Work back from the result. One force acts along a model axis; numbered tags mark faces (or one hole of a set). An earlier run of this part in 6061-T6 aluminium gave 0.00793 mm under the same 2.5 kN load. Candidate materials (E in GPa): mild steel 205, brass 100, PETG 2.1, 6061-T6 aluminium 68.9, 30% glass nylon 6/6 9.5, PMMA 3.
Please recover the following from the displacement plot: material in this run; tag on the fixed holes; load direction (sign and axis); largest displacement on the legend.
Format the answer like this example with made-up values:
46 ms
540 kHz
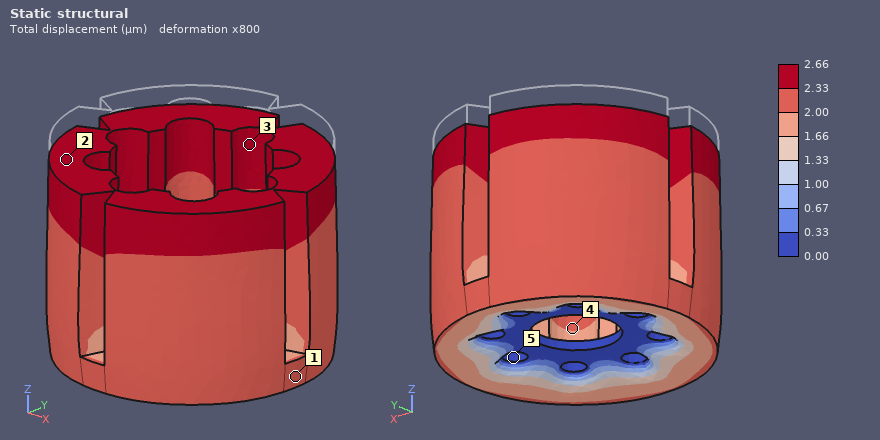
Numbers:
mild steel
5
-Z
2.66 µm
